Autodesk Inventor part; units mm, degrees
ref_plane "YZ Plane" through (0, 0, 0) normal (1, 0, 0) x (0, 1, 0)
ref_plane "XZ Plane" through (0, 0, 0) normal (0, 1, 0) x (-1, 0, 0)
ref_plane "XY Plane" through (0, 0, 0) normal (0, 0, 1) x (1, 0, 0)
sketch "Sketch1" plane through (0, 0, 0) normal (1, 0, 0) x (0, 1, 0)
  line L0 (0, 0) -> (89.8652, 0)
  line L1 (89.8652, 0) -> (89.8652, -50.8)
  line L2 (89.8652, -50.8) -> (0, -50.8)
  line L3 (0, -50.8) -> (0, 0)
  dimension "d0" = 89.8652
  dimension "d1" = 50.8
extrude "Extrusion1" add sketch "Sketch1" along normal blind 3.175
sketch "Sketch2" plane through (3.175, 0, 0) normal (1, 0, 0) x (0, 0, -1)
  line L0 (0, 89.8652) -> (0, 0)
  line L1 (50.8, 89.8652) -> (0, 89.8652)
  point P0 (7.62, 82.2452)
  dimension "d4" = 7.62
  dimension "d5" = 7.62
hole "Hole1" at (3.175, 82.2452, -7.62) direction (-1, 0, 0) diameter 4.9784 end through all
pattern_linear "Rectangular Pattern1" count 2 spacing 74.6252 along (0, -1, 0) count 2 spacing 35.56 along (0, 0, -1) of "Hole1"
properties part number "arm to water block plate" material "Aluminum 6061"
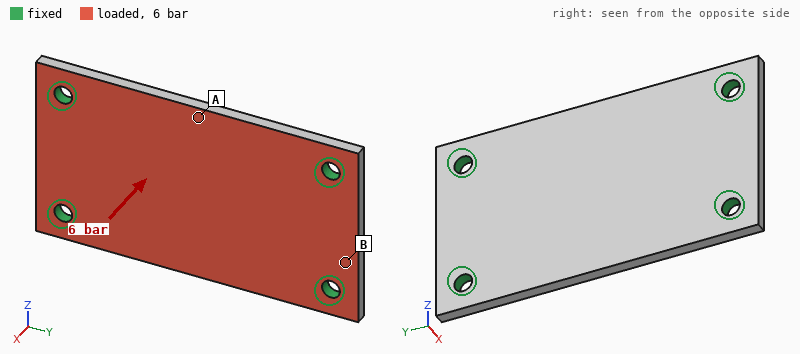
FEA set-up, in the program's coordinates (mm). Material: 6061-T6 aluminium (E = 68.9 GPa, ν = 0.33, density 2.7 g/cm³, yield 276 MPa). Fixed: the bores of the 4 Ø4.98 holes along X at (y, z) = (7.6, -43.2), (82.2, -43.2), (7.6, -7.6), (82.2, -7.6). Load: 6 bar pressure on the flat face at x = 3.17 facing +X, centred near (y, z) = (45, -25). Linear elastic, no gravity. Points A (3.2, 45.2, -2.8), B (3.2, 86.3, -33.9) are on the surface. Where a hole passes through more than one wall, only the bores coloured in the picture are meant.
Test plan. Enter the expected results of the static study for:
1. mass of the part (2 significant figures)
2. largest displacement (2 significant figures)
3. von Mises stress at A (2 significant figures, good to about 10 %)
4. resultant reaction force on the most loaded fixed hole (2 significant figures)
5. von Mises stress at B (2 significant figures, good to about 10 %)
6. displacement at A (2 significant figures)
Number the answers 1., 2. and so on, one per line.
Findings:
1. 38 g
2. 0.27 mm
3. 87 MPa
4. 670 N
5. 38 MPa
6. 0.27 mm
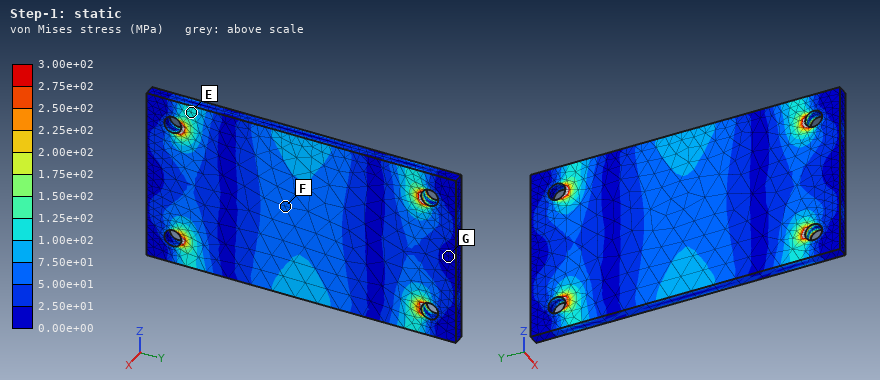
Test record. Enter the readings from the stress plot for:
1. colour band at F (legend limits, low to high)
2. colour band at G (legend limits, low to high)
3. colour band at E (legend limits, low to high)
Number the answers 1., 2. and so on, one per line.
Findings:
1. 5.00e+01 to 7.50e+01 MPa
2. 0.00e+00 to 2.50e+01 MPa
3. 1.00e+02 to 1.25e+02 MPa
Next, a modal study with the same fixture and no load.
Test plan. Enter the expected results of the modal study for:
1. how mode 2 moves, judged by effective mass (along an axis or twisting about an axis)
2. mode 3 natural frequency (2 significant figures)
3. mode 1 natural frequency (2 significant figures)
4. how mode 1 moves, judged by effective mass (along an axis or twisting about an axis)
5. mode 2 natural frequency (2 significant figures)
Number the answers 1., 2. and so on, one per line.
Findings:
1. twisting about Y
2. 7800 Hz
3. 2900 Hz
4. along X
5. 4300 Hz
